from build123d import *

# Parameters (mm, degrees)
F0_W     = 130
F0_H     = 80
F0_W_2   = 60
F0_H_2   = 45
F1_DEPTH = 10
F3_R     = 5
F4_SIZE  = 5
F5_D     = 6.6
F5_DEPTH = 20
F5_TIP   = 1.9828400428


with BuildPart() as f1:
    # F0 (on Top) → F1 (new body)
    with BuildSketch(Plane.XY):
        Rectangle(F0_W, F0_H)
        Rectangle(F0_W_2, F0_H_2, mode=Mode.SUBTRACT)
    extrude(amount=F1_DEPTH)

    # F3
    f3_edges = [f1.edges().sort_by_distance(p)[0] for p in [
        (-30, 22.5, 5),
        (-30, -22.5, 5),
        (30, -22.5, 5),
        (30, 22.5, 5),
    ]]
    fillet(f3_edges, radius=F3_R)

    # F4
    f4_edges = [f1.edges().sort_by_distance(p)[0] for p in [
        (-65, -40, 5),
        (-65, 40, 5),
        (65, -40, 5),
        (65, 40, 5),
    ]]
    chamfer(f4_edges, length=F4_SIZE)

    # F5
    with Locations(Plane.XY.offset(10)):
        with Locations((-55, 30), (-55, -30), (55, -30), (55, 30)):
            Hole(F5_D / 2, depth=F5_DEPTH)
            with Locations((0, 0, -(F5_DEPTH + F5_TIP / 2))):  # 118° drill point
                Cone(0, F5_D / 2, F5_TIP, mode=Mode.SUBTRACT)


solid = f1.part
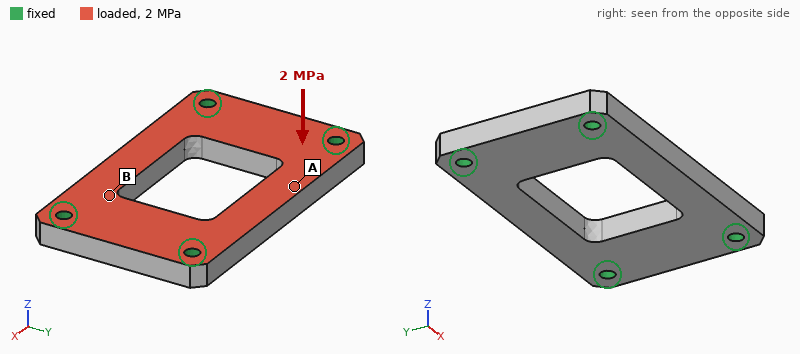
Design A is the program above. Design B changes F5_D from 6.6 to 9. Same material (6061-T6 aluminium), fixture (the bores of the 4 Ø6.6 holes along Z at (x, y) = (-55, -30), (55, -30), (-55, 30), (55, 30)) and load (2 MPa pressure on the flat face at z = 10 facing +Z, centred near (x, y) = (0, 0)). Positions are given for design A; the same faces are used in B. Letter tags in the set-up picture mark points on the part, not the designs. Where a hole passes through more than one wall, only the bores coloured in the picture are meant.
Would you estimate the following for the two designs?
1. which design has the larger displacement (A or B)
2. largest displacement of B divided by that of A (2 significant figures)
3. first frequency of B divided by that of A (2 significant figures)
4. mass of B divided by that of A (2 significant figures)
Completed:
A
0.86
1.1
0.98
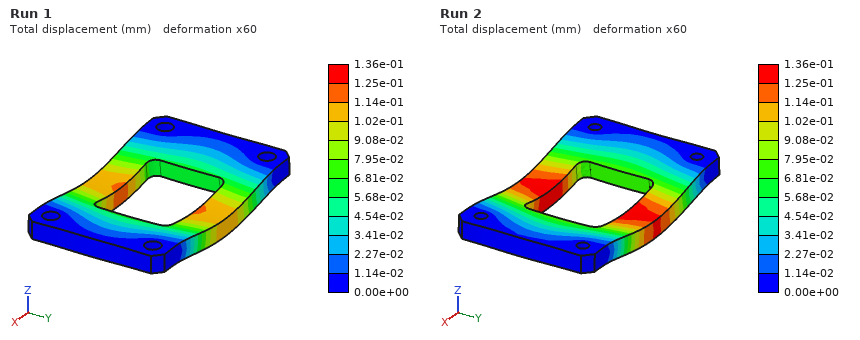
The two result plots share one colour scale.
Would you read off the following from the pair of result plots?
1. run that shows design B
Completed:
Run 1
